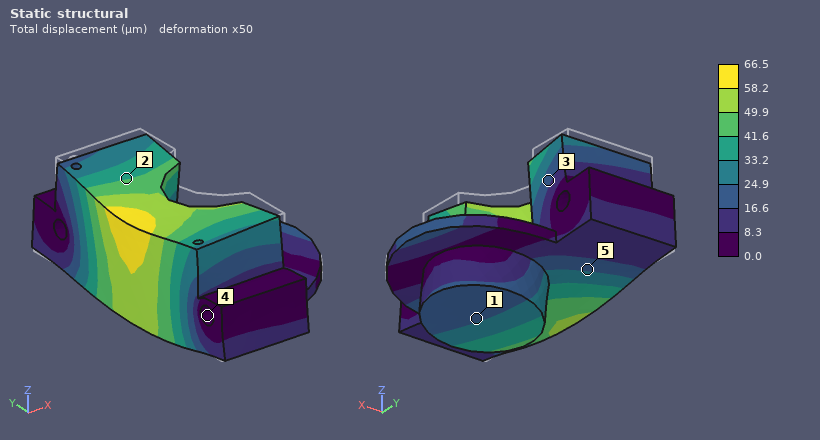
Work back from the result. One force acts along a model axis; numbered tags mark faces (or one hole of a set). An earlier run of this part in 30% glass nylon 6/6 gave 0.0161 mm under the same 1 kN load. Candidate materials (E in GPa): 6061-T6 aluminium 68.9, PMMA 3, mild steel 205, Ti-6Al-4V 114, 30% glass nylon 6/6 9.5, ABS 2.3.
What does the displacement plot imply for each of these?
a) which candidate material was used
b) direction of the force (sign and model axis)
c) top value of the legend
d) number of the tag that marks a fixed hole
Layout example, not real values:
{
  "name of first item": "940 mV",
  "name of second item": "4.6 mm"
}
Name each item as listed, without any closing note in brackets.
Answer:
{
  "which candidate material was used": "ABS",
  "direction of the force": "-Z",
  "top value of the legend": "66.5 µm",
  "number of the tag that marks a fixed hole": "4"
}
